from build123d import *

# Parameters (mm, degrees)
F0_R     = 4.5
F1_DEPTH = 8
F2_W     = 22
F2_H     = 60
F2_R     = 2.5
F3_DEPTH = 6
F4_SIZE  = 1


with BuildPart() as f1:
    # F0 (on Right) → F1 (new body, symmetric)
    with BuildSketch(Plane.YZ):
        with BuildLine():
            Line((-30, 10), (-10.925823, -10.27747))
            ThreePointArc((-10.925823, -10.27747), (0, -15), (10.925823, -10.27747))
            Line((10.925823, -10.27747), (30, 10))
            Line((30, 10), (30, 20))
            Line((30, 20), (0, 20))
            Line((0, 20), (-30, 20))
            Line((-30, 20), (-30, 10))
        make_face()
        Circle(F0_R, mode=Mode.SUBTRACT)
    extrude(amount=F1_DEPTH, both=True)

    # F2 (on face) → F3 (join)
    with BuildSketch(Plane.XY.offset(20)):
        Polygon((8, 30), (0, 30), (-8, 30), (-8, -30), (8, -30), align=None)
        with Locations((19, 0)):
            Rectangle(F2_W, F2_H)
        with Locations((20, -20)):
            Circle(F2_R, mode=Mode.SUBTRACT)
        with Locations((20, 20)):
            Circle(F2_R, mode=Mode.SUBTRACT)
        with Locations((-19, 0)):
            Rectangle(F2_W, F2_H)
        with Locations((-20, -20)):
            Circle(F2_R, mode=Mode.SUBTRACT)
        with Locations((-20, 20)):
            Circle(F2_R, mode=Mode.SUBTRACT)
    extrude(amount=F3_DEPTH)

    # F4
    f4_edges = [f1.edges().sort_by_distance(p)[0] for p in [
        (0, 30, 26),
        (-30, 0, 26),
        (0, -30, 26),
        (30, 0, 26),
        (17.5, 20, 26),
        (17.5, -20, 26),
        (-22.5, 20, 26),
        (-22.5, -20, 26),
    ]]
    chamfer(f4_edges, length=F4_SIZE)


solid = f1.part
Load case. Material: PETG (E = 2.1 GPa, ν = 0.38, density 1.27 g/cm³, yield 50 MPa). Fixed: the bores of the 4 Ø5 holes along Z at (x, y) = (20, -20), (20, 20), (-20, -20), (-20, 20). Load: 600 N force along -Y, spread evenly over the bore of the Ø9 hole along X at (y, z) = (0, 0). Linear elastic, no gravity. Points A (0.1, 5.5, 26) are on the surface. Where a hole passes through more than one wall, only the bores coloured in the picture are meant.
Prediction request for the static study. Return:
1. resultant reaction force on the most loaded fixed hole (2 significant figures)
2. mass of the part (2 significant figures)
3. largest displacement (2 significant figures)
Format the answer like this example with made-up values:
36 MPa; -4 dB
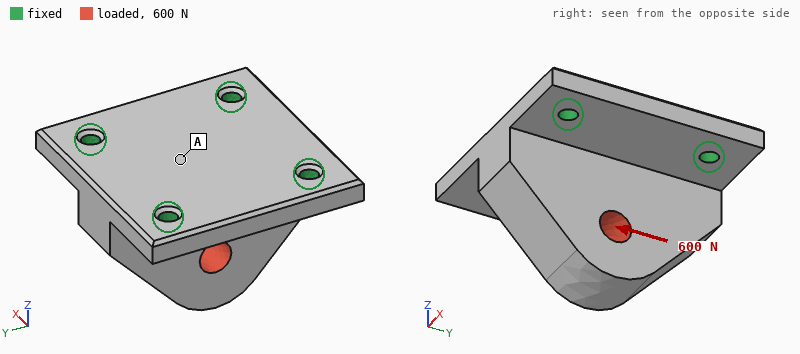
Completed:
230 N; 56 g; 0.20 mm
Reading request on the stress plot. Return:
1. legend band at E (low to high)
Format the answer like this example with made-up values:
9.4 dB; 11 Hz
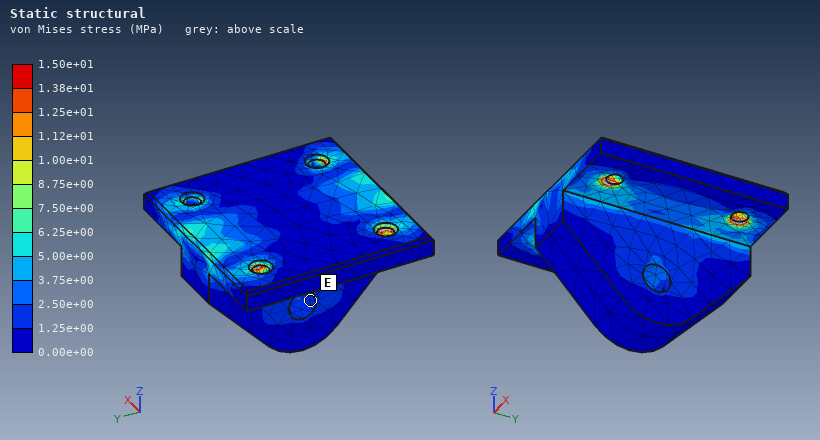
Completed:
1.25e+00 to 2.50e+00 MPa
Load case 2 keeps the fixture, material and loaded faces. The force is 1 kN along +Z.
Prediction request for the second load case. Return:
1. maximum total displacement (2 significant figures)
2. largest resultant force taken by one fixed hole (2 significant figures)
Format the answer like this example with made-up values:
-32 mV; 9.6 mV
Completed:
0.15 mm; 260 N
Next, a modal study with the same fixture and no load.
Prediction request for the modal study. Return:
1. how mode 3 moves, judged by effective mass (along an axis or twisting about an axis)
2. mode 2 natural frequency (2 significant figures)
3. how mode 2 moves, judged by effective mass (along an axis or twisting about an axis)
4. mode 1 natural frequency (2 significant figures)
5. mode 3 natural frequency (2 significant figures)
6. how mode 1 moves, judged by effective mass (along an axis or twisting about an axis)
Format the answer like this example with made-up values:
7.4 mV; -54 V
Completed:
along Z; 1900 Hz; along Y; 1700 Hz; 2200 Hz; along X
